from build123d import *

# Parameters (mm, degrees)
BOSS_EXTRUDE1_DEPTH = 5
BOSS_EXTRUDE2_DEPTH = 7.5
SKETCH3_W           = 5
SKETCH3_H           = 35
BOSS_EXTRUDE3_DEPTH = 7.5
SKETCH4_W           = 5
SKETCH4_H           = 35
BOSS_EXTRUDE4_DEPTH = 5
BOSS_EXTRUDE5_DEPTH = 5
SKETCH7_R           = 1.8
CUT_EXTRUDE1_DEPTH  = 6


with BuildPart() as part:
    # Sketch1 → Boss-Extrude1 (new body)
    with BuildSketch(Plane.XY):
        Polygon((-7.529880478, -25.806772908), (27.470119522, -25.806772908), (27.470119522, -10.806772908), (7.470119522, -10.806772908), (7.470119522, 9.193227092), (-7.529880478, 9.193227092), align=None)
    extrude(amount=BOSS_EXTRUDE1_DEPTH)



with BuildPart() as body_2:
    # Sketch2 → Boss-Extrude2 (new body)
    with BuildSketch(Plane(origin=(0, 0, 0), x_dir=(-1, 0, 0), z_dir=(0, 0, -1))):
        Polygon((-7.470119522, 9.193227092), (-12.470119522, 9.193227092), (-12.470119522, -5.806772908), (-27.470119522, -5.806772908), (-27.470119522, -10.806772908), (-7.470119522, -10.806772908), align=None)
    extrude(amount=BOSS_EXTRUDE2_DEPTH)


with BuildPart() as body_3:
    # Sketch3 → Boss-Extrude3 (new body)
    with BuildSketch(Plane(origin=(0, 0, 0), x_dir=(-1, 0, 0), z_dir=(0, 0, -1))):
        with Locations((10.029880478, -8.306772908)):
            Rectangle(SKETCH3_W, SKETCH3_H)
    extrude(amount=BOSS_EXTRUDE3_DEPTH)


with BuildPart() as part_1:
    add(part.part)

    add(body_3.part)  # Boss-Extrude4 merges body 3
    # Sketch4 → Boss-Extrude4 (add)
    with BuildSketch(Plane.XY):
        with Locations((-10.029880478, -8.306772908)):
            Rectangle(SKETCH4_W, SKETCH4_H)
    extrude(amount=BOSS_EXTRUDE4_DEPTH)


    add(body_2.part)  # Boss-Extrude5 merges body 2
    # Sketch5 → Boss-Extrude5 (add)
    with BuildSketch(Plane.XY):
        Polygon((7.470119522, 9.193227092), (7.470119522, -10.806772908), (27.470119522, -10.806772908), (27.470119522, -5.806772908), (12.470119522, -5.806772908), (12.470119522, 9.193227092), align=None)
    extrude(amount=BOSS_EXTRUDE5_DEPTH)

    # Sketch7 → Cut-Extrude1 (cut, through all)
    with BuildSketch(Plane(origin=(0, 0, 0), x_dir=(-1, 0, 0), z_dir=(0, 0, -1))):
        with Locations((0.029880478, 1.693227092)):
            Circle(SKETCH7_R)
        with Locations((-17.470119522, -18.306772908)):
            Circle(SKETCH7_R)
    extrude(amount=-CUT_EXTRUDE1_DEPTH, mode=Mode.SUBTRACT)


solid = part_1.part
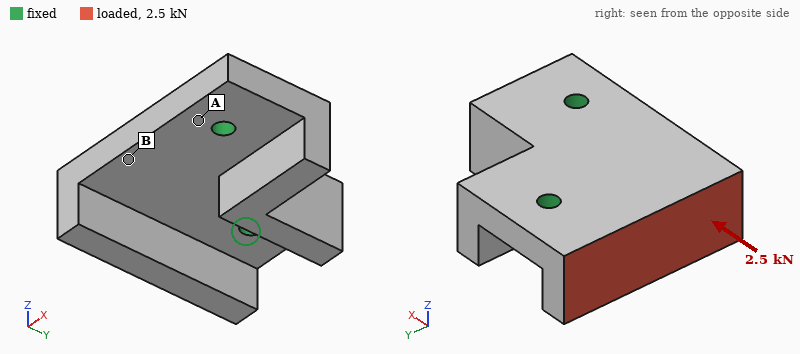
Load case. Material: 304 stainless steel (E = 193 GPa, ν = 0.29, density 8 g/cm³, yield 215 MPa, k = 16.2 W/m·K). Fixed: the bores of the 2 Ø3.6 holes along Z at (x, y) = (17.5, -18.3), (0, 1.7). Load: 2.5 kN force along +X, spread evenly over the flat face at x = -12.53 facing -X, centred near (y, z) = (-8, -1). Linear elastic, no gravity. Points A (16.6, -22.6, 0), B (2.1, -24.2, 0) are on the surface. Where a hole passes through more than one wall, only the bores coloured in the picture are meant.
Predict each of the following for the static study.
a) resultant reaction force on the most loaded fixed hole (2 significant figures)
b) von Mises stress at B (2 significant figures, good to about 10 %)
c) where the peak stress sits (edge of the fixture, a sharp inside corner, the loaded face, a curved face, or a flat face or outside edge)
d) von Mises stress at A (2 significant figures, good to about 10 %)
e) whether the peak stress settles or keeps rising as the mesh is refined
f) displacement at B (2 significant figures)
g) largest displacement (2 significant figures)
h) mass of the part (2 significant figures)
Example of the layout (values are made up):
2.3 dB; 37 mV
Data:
1.3 kN; 53 MPa; edge of the fixture; 16 MPa; keeps rising; 5.2 µm; 33 µm; 67 g
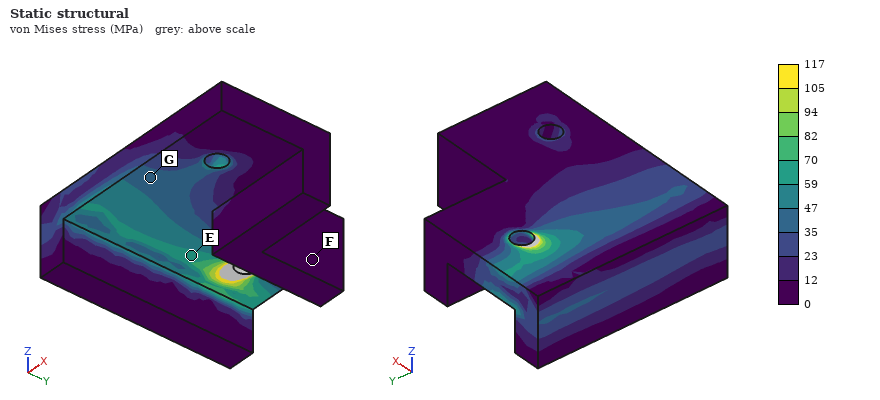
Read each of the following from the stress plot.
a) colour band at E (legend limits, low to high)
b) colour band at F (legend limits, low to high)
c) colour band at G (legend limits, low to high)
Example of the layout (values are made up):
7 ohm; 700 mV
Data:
59 to 70 MPa; 0 to 12 MPa; 35 to 47 MPa
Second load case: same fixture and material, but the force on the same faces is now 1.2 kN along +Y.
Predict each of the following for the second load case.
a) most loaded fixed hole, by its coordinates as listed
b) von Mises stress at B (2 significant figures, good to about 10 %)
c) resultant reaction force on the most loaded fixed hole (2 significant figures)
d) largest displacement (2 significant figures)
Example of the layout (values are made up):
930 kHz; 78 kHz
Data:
(0, 1.7); 12 MPa; 1.4 kN; 13 µm
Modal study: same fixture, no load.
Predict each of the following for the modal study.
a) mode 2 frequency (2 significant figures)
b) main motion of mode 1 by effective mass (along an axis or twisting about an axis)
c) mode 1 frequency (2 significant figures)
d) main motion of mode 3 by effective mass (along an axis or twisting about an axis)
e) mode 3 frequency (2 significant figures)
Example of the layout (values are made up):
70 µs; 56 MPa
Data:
13 kHz; along Z; 6100 Hz; along Z; 15 kHz
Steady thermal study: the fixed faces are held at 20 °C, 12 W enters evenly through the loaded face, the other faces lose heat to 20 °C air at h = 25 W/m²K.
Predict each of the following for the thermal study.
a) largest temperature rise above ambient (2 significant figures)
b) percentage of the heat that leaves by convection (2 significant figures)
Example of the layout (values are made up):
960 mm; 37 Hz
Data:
75 K; 19 %
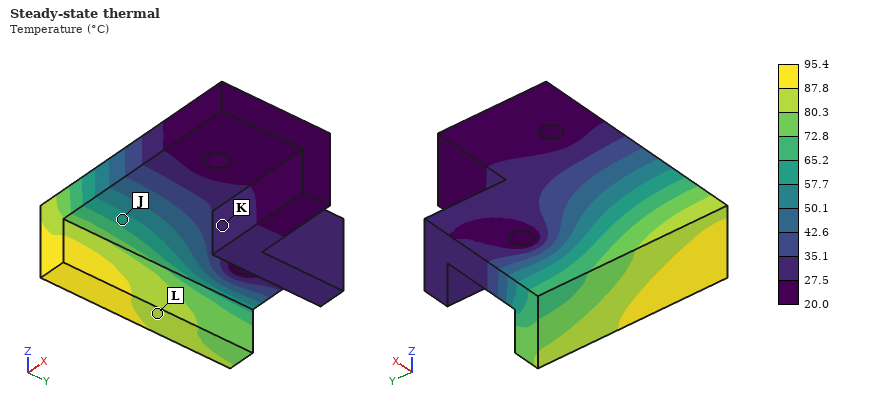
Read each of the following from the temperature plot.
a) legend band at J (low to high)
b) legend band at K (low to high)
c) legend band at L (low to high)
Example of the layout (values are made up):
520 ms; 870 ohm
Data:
57.7 to 65.2 °C; 27.5 to 35.1 °C; 80.3 to 87.8 °C
